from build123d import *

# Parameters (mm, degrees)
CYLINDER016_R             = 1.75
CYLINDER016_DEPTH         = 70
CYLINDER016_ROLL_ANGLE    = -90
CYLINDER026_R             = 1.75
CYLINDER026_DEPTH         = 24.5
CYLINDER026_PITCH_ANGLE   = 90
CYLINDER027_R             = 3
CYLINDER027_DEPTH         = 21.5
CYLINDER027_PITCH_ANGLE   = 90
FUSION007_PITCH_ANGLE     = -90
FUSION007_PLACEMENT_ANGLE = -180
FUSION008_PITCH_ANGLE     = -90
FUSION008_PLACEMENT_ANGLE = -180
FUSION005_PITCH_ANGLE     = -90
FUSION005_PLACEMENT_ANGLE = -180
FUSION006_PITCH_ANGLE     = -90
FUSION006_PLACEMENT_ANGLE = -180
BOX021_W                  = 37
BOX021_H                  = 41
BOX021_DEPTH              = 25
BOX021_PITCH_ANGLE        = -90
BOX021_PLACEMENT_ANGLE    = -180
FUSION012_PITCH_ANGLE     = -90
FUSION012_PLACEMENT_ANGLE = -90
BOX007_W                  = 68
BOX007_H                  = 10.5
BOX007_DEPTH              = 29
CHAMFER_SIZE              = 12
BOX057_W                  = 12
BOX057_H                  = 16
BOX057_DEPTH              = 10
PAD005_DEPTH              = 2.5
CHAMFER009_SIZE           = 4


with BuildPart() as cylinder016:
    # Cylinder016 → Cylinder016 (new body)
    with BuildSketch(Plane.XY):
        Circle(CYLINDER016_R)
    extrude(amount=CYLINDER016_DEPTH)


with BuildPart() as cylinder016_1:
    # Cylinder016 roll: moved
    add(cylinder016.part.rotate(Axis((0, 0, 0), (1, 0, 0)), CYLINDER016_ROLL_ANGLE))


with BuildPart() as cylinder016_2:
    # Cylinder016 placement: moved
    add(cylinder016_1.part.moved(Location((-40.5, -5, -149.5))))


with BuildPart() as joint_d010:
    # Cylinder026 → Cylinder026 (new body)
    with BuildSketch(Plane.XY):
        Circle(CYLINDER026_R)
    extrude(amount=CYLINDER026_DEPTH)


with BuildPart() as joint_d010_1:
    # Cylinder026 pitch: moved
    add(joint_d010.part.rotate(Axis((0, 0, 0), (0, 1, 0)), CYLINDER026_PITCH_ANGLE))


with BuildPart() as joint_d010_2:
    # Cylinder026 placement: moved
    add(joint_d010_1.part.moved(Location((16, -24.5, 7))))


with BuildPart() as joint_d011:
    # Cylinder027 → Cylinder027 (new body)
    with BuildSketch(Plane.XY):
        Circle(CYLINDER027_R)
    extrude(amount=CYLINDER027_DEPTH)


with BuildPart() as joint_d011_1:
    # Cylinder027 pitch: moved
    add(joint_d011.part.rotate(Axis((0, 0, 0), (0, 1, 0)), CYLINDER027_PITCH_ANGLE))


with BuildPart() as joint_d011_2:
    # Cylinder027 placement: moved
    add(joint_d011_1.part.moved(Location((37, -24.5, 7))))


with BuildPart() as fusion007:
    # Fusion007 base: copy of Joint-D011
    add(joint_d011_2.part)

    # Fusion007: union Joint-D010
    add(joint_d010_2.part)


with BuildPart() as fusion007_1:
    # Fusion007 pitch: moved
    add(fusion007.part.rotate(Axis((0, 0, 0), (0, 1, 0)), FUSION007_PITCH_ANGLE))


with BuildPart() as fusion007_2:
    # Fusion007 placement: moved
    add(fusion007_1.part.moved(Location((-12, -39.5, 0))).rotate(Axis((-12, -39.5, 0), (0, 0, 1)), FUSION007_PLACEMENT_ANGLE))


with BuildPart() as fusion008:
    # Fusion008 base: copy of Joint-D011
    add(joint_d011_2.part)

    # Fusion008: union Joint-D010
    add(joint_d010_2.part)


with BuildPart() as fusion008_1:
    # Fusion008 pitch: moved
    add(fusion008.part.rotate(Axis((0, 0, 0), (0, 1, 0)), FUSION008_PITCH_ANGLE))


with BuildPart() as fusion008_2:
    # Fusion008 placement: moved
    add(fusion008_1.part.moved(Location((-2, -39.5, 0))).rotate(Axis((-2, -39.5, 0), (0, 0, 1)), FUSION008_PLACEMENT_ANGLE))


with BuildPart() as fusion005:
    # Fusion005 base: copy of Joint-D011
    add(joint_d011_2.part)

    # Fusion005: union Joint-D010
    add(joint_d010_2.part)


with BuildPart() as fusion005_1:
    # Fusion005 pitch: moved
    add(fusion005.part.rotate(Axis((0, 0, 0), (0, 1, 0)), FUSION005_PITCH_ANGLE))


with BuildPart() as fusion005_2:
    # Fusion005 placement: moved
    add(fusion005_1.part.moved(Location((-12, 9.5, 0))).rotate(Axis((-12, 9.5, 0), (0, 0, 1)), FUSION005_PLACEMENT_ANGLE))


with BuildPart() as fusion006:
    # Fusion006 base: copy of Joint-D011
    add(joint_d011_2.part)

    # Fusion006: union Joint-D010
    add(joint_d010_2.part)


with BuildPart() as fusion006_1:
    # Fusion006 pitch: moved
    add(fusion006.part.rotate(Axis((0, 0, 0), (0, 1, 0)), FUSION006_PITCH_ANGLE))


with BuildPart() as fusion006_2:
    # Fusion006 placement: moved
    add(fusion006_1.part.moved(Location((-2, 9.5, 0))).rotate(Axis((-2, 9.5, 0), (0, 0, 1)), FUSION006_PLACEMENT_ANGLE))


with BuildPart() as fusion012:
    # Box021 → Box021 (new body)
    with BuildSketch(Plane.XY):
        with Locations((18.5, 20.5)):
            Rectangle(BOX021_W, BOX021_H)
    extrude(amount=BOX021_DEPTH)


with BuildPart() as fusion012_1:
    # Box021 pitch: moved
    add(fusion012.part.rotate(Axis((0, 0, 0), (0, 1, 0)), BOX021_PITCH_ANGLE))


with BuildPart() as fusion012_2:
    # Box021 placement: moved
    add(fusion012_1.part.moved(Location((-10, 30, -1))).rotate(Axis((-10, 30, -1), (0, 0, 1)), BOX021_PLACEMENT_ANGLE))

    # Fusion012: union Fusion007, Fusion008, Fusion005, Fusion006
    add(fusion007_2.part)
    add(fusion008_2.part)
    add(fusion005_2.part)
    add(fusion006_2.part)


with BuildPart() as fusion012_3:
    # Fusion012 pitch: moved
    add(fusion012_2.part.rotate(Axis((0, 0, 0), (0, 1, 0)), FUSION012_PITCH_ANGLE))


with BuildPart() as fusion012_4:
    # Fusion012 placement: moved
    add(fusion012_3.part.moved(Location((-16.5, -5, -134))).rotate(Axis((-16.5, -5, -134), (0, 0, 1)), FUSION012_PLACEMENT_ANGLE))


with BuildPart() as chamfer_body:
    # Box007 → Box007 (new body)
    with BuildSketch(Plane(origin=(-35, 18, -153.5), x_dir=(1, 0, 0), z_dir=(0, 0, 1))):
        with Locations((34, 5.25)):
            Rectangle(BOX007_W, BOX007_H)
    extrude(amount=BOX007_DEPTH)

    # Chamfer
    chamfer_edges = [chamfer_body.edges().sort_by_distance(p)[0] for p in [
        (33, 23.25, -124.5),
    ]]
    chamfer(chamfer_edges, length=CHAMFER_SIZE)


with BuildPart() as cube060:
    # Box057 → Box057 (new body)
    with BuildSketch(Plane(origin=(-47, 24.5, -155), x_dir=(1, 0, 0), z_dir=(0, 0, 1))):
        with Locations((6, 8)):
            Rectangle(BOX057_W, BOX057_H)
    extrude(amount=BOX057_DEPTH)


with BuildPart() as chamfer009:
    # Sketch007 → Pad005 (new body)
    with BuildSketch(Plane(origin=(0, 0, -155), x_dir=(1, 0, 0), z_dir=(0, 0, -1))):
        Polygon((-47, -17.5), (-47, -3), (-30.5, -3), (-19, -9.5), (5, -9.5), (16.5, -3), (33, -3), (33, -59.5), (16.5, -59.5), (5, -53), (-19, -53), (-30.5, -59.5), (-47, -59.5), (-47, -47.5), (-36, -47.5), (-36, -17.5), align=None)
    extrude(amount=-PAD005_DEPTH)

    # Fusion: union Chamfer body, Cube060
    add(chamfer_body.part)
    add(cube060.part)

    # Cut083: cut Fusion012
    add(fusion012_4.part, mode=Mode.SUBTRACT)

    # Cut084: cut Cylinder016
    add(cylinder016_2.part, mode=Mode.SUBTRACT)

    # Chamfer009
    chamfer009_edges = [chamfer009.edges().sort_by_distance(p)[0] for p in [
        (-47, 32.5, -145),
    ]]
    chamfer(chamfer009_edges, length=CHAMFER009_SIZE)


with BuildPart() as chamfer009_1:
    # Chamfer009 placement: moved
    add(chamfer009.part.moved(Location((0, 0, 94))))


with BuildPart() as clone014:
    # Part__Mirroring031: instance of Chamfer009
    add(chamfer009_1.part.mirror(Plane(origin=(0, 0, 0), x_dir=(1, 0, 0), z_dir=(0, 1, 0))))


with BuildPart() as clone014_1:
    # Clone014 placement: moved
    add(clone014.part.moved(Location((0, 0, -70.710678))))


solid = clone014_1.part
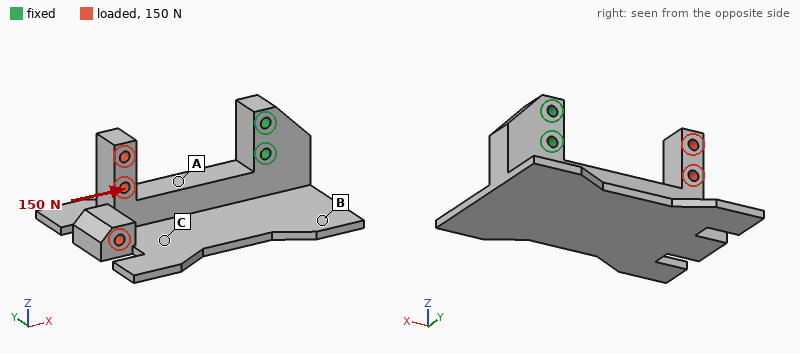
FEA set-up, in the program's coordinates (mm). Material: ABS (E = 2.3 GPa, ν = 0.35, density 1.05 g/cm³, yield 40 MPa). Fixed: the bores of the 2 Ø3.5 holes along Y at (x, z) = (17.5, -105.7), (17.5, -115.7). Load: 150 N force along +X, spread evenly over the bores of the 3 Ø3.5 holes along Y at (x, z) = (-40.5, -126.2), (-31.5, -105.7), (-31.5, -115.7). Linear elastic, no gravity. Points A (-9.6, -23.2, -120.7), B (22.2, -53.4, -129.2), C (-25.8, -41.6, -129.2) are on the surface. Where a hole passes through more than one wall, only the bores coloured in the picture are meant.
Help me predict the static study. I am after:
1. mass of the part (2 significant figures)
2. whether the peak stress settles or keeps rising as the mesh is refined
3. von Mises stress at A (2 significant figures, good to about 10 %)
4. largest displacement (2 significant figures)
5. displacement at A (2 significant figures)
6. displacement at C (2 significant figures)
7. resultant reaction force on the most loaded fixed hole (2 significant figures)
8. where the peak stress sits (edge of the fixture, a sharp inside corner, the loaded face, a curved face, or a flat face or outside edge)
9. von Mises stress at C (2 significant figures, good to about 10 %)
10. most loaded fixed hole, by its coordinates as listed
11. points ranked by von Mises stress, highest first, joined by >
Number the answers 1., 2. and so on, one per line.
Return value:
1. 22 g
2. keeps rising
3. 6.6 MPa
4. 0.92 mm
5. 0.17 mm
6. 0.38 mm
7. 150 N
8. edge of the fixture
9. 1.6 MPa
10. (17.5, -115.7)
11. A > C > B
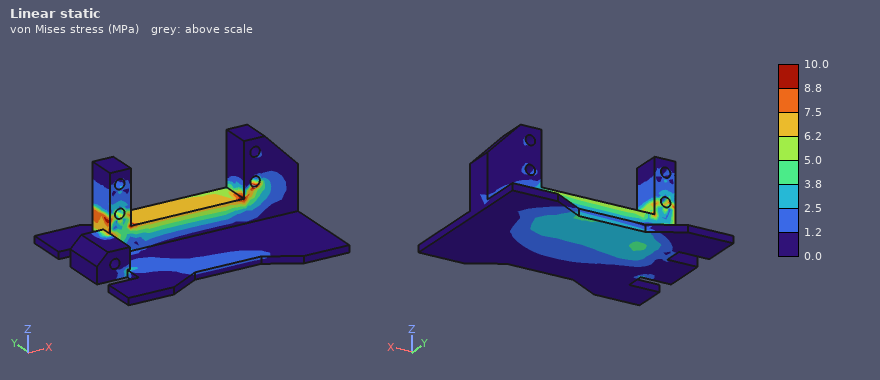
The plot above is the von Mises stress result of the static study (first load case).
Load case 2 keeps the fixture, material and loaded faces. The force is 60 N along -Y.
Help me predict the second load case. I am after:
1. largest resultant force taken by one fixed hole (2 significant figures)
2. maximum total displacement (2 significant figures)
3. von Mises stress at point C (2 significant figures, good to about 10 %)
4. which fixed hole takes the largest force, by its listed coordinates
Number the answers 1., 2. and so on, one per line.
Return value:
1. 65 N
2. 1.2 mm
3. 2.1 MPa
4. (17.5, -115.7)
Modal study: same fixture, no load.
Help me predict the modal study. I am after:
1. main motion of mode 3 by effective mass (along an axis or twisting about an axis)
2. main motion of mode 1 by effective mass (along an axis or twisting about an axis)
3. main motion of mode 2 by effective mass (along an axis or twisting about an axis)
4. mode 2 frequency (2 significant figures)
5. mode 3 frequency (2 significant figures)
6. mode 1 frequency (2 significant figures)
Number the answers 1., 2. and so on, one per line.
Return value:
1. twisting about X
2. along Z
3. along Y
4. 460 Hz
5. 610 Hz
6. 390 Hz
